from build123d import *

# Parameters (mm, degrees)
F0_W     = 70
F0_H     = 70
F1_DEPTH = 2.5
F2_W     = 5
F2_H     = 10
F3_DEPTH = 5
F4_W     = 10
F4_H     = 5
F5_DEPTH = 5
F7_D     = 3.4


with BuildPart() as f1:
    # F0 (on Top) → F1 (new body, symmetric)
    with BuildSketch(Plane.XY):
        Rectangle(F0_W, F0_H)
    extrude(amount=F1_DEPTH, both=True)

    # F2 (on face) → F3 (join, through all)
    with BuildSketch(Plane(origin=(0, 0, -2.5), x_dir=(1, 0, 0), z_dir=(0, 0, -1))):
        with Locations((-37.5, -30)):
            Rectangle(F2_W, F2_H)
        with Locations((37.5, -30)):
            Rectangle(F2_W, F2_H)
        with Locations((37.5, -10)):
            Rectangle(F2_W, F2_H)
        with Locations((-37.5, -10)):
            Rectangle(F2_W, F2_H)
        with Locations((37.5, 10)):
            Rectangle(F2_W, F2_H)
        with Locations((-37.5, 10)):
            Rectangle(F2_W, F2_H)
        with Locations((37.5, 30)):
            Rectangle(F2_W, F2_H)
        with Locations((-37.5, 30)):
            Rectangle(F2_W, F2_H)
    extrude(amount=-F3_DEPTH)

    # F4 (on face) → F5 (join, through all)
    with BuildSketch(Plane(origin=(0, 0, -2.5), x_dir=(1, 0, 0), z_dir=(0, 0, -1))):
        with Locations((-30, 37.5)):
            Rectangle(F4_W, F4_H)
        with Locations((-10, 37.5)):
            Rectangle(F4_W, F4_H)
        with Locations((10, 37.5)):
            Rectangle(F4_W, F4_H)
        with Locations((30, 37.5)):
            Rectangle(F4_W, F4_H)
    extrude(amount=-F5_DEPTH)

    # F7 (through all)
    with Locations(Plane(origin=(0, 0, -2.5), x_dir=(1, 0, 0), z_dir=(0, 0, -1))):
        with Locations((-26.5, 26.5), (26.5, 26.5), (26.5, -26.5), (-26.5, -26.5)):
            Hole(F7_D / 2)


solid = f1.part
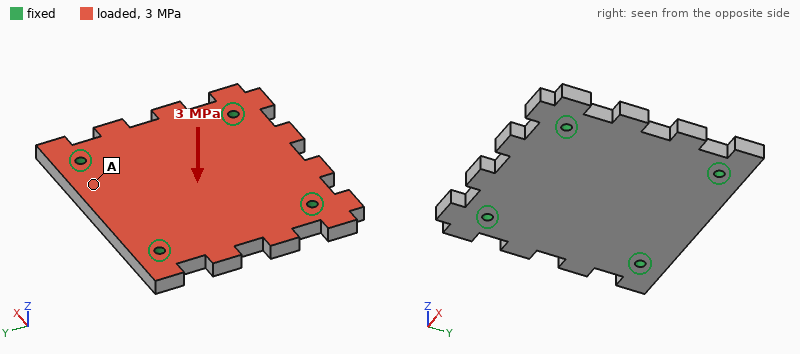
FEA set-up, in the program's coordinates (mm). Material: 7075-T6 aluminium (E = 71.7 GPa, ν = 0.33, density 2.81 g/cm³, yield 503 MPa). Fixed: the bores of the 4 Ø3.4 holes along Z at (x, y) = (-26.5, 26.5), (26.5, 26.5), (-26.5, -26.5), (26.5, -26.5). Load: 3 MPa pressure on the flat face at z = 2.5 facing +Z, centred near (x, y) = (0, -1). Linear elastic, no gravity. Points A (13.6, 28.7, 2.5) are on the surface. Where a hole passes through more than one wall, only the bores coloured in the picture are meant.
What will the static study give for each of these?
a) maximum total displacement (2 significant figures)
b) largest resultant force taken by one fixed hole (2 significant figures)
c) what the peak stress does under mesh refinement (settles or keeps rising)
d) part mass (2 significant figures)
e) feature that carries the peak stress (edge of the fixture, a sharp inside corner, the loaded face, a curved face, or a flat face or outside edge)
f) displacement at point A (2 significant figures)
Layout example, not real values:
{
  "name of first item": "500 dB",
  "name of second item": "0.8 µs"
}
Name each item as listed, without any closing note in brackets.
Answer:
{
  "maximum total displacement": "0.23 mm",
  "largest resultant force taken by one fixed hole": "4.3 kN",
  "what the peak stress does under mesh refinement": "keeps rising",
  "part mass": "77 g",
  "feature that carries the peak stress": "edge of the fixture",
  "displacement at point A": "0.070 mm"
}
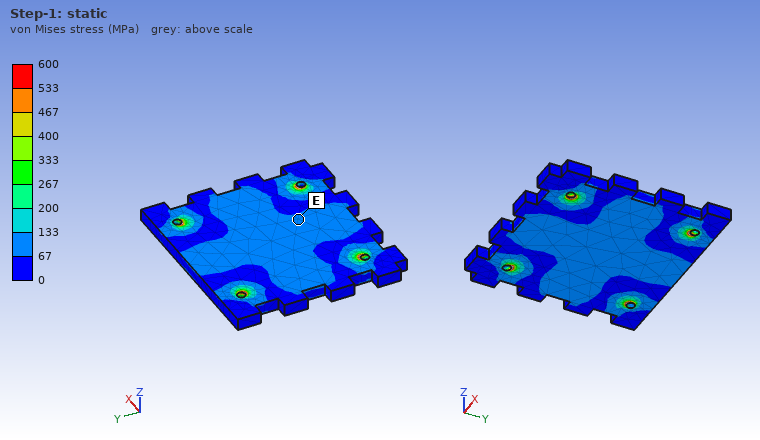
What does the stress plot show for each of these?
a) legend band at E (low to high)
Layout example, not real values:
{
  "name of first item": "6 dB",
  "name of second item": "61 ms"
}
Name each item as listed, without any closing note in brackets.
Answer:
{
  "legend band at E": "67 to 133 MPa"
}
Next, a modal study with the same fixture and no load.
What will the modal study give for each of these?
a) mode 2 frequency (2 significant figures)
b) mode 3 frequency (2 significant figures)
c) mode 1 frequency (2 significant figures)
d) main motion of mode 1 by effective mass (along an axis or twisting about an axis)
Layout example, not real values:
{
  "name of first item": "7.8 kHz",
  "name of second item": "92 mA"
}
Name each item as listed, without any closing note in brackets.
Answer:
{
  "mode 2 frequency": "8000 Hz",
  "mode 3 frequency": "8200 Hz",
  "mode 1 frequency": "5900 Hz",
  "main motion of mode 1 by effective mass": "along Z"
}
